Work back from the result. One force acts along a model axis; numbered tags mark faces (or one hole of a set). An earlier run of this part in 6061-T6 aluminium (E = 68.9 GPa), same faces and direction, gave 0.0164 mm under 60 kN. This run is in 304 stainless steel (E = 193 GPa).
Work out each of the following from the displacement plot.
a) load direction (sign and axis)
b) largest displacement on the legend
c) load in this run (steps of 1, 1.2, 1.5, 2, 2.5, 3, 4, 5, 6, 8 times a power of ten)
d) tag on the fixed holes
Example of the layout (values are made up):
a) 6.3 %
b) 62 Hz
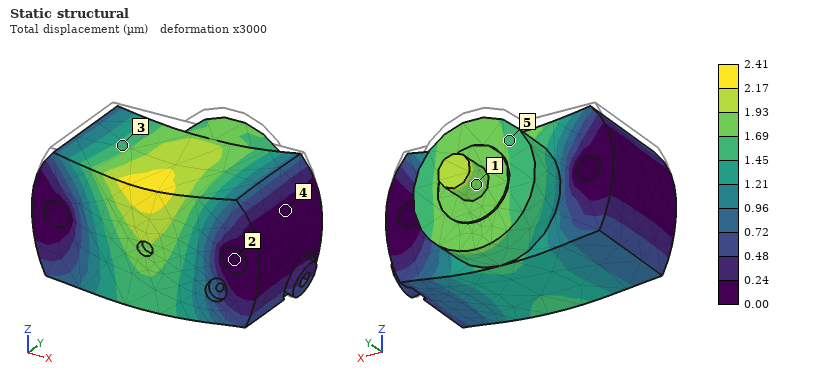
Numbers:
a) -Z
b) 2.41 µm
c) 25 kN
d) 2
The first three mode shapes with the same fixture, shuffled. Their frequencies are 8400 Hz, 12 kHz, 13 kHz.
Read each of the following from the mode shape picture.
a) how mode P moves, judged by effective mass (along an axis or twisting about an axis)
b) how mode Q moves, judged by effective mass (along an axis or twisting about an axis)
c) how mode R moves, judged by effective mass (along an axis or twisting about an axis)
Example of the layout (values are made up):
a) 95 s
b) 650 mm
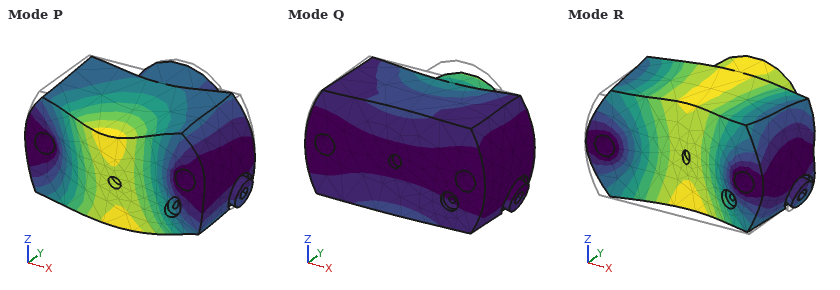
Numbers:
a) along Z
b) along Z
c) along Y
